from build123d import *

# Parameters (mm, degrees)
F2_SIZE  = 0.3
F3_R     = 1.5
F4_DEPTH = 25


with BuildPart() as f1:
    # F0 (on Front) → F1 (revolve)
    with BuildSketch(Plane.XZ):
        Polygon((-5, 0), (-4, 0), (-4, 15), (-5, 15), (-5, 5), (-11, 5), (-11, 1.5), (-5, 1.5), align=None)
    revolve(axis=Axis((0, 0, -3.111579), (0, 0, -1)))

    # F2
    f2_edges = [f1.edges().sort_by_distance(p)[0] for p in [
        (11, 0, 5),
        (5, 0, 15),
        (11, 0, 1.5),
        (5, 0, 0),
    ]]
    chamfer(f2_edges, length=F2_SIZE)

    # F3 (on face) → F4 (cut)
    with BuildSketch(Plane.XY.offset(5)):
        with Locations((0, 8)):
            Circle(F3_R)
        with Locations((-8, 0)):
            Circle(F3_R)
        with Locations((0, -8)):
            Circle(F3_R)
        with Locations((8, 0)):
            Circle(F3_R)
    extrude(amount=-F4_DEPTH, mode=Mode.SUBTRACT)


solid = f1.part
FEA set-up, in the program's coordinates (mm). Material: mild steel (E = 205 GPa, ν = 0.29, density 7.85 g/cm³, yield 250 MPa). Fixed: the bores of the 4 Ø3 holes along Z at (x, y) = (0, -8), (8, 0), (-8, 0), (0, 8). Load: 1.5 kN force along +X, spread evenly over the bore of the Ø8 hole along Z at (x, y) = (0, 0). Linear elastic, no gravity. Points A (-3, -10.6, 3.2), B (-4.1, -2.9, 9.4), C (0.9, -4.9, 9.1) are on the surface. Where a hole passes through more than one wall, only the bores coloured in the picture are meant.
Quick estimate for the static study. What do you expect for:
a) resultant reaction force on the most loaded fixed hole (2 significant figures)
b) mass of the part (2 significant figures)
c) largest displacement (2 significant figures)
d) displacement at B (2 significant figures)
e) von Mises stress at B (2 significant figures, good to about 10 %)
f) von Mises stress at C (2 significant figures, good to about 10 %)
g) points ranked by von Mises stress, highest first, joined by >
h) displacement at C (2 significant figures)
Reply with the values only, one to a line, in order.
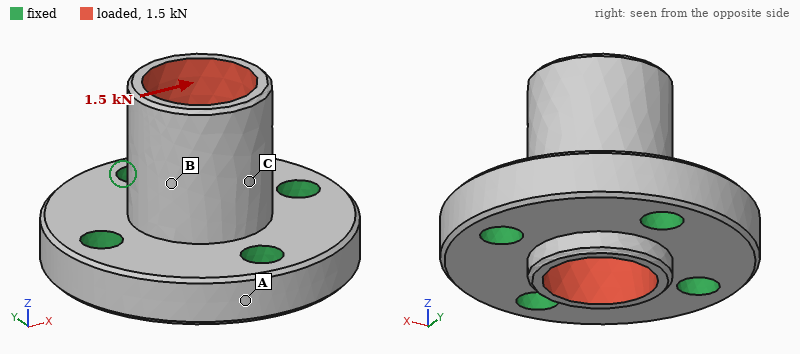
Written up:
620 N
11 g
9.9 µm
5.7 µm
43 MPa
63 MPa
C > B > A
4.7 µm
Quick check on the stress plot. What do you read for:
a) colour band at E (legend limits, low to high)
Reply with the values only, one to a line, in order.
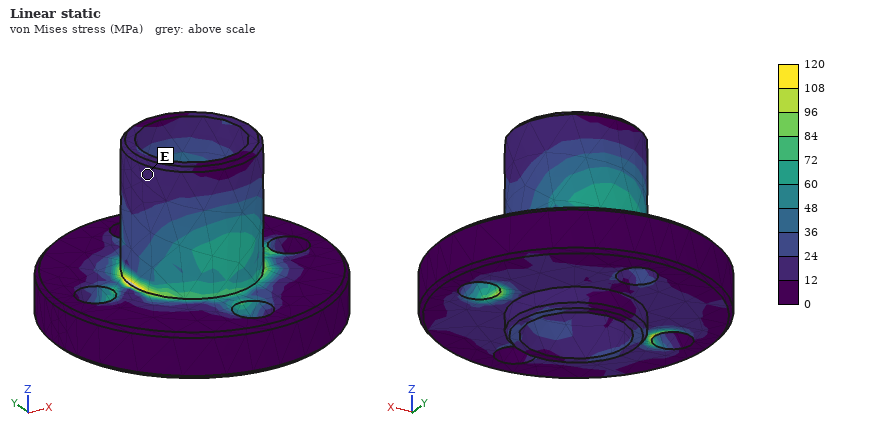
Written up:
12 to 24 MPa
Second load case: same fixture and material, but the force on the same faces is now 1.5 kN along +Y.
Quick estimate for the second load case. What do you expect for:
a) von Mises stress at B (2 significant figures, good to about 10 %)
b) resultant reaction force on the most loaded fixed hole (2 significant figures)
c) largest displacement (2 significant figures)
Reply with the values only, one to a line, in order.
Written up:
55 MPa
620 N
9.9 µm
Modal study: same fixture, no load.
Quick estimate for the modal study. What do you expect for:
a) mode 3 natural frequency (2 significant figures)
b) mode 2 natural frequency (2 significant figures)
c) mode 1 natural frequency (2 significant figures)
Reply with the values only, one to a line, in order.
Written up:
40 kHz
40 kHz
40 kHz
